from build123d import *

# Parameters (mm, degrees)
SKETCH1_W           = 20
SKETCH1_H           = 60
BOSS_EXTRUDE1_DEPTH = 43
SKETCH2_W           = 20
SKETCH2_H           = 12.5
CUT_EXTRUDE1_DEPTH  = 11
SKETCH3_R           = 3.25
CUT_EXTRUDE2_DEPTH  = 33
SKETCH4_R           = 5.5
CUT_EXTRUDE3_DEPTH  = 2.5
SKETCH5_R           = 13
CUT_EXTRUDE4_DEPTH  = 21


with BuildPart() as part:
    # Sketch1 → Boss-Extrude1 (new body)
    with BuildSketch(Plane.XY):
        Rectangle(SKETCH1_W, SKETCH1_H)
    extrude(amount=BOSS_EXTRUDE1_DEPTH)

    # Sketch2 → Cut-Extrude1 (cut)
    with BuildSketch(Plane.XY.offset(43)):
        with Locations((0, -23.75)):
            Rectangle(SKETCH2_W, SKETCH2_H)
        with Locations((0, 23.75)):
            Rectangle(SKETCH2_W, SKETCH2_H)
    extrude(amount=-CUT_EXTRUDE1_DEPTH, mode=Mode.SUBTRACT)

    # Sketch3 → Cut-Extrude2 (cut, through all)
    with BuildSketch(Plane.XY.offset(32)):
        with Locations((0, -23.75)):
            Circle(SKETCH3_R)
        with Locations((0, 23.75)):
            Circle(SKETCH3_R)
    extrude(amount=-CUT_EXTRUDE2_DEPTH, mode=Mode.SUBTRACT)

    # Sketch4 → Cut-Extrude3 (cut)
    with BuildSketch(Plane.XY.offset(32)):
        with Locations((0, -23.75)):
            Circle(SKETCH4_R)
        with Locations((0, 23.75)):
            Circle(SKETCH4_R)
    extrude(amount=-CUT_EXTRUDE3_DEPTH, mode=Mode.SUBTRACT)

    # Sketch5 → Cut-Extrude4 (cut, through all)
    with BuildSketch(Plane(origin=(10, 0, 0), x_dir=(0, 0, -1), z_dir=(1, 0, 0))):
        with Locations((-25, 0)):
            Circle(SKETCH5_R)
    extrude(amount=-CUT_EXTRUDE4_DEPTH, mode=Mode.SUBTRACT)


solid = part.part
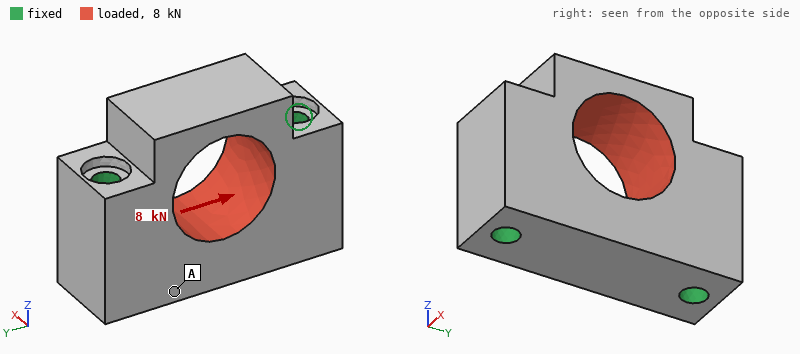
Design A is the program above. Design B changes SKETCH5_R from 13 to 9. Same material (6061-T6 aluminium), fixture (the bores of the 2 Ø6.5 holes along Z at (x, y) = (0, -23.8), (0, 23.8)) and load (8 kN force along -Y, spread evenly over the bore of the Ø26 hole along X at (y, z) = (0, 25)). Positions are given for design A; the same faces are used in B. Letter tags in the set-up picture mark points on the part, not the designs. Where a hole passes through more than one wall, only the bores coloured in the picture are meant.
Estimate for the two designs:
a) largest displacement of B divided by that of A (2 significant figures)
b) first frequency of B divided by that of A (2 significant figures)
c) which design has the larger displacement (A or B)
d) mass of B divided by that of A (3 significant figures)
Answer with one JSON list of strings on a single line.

["0.49", "0.99", "A", "1.17"]
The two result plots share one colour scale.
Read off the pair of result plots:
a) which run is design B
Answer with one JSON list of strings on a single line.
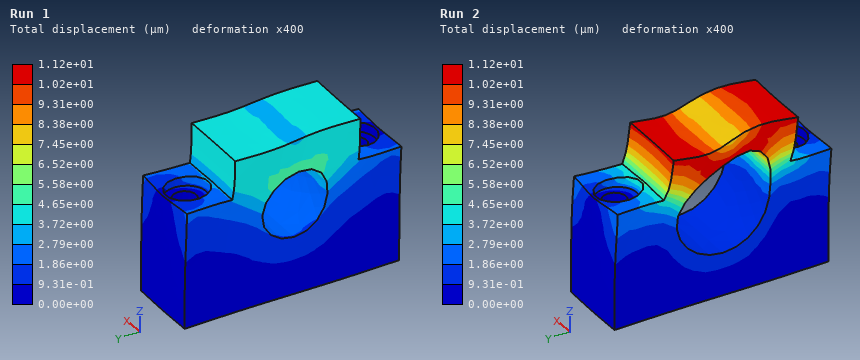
["Run 1"]
